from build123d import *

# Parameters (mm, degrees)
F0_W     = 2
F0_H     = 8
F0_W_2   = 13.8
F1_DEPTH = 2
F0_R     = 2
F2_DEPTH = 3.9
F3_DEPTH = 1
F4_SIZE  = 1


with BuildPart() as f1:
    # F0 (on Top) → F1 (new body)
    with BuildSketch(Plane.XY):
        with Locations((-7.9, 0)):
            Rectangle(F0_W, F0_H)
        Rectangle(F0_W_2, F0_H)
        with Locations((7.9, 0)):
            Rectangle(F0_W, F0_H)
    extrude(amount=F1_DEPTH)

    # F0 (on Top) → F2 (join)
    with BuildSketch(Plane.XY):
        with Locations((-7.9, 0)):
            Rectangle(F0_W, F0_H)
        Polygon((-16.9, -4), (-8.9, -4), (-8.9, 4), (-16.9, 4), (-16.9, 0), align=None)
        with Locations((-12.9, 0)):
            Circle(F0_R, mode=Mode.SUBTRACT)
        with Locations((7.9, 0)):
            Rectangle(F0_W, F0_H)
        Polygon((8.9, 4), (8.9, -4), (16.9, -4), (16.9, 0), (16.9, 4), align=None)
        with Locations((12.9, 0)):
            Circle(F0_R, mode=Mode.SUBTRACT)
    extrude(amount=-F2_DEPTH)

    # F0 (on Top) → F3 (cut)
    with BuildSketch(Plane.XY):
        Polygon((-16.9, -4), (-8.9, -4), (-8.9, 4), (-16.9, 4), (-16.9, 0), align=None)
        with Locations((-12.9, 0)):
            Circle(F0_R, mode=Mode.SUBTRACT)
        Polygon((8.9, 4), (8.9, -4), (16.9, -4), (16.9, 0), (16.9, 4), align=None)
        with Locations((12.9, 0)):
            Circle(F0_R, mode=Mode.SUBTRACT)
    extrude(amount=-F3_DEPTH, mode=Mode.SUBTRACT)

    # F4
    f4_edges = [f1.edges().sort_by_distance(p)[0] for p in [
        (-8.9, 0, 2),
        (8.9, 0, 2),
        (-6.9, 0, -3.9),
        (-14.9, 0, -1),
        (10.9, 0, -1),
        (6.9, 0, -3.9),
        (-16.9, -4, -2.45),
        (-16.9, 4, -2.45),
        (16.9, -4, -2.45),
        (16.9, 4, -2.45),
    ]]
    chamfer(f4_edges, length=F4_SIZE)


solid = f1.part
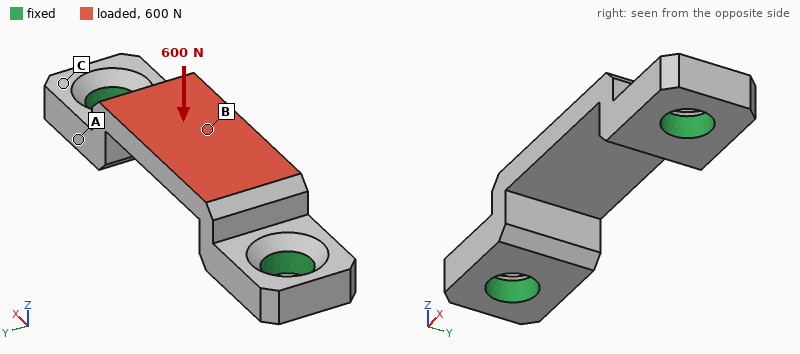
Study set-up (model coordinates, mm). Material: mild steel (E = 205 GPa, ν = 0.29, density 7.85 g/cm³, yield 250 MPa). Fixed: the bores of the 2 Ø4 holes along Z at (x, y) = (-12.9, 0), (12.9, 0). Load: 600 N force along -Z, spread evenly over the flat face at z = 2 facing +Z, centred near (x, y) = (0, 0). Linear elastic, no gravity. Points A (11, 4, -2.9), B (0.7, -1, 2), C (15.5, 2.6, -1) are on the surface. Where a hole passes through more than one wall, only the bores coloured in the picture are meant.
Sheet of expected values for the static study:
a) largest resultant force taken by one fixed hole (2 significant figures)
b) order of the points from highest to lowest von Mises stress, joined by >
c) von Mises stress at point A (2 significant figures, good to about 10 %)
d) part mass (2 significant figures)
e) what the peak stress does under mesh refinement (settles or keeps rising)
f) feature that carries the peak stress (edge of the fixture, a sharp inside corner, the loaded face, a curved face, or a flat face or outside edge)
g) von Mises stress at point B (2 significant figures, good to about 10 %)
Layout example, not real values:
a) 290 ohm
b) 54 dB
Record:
a) 470 N
b) B > A > C
c) 17 MPa
d) 5.3 g
e) keeps rising
f) edge of the fixture
g) 96 MPa
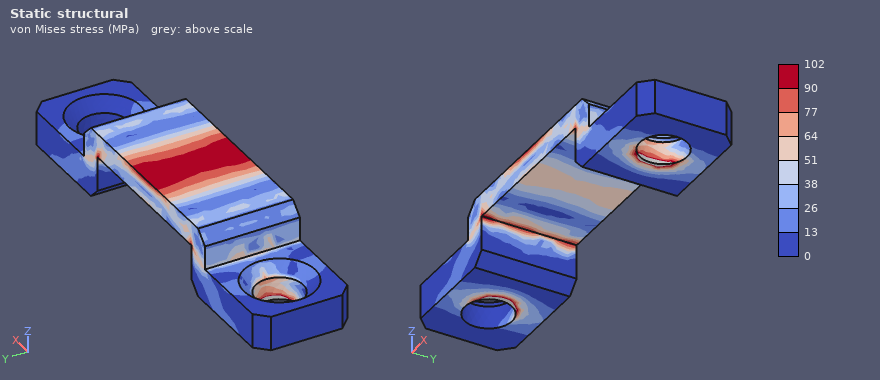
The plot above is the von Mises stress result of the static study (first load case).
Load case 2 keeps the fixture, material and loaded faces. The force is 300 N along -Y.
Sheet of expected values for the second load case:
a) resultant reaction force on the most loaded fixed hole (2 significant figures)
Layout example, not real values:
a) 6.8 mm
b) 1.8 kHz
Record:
a) 150 N
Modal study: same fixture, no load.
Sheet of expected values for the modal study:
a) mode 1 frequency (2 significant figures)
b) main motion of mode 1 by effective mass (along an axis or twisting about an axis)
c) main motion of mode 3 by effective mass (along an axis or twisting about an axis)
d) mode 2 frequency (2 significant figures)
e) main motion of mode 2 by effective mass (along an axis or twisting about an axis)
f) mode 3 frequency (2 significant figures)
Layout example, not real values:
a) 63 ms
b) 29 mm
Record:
a) 29 kHz
b) along Y
c) along X
d) 32 kHz
e) along Z
f) 35 kHz
